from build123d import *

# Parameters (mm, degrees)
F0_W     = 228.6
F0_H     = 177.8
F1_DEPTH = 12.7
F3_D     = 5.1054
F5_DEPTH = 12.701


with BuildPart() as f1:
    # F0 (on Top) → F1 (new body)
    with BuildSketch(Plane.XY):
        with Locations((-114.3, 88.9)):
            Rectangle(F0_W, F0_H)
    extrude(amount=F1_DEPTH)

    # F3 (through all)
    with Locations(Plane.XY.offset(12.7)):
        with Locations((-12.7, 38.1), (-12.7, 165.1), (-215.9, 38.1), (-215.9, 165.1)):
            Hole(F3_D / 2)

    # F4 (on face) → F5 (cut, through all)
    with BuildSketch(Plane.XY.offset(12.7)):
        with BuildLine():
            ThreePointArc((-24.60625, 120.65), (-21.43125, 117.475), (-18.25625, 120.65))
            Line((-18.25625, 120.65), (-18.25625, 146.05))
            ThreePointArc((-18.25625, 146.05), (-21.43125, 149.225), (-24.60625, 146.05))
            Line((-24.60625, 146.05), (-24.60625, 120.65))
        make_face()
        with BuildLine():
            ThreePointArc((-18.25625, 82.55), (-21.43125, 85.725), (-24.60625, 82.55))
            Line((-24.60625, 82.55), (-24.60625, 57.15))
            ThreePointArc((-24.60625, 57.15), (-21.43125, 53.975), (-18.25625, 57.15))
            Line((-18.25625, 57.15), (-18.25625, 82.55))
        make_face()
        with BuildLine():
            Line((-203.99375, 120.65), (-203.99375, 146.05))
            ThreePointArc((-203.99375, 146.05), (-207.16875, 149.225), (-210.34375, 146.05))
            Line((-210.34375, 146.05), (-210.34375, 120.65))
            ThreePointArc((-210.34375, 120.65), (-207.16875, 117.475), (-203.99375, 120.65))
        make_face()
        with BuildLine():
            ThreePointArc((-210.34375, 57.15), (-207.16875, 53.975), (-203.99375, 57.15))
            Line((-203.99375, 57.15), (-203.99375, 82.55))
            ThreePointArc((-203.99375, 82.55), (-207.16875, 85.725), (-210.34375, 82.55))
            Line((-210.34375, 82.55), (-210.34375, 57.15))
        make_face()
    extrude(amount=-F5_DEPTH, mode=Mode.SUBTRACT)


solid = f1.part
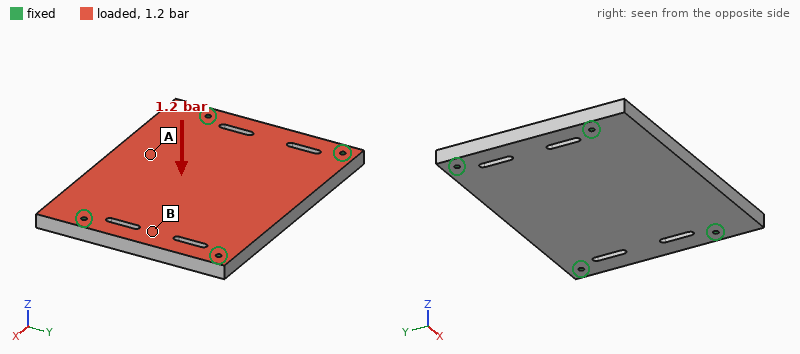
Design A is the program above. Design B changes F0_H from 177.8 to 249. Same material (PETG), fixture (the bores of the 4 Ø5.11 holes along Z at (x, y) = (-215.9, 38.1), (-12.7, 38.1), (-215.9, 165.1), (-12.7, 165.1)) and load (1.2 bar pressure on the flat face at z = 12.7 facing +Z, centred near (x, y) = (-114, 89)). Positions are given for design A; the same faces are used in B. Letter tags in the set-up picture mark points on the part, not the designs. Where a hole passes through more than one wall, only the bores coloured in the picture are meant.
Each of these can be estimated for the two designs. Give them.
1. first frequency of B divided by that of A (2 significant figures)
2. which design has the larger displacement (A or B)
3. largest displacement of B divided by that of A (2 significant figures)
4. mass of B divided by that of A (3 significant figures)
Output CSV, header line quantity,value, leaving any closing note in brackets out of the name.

quantity,value
first frequency of B divided by that of A,0.81
which design has the larger displacement,B
largest displacement of B divided by that of A,2.0
mass of B divided by that of A,1.41
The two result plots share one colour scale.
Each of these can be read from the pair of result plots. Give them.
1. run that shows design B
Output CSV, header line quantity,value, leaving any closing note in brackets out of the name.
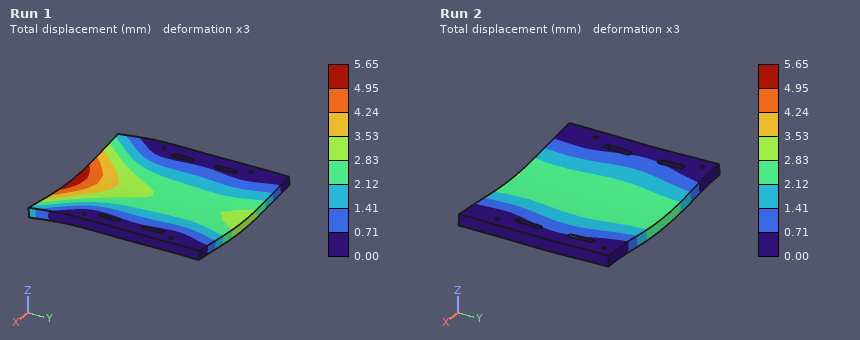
quantity,value
run that shows design B,Run 1
